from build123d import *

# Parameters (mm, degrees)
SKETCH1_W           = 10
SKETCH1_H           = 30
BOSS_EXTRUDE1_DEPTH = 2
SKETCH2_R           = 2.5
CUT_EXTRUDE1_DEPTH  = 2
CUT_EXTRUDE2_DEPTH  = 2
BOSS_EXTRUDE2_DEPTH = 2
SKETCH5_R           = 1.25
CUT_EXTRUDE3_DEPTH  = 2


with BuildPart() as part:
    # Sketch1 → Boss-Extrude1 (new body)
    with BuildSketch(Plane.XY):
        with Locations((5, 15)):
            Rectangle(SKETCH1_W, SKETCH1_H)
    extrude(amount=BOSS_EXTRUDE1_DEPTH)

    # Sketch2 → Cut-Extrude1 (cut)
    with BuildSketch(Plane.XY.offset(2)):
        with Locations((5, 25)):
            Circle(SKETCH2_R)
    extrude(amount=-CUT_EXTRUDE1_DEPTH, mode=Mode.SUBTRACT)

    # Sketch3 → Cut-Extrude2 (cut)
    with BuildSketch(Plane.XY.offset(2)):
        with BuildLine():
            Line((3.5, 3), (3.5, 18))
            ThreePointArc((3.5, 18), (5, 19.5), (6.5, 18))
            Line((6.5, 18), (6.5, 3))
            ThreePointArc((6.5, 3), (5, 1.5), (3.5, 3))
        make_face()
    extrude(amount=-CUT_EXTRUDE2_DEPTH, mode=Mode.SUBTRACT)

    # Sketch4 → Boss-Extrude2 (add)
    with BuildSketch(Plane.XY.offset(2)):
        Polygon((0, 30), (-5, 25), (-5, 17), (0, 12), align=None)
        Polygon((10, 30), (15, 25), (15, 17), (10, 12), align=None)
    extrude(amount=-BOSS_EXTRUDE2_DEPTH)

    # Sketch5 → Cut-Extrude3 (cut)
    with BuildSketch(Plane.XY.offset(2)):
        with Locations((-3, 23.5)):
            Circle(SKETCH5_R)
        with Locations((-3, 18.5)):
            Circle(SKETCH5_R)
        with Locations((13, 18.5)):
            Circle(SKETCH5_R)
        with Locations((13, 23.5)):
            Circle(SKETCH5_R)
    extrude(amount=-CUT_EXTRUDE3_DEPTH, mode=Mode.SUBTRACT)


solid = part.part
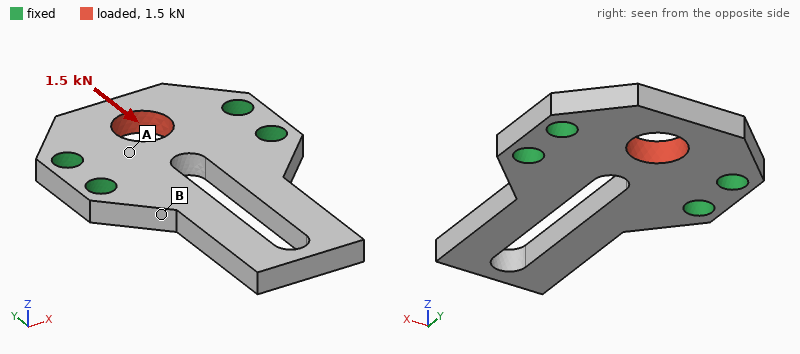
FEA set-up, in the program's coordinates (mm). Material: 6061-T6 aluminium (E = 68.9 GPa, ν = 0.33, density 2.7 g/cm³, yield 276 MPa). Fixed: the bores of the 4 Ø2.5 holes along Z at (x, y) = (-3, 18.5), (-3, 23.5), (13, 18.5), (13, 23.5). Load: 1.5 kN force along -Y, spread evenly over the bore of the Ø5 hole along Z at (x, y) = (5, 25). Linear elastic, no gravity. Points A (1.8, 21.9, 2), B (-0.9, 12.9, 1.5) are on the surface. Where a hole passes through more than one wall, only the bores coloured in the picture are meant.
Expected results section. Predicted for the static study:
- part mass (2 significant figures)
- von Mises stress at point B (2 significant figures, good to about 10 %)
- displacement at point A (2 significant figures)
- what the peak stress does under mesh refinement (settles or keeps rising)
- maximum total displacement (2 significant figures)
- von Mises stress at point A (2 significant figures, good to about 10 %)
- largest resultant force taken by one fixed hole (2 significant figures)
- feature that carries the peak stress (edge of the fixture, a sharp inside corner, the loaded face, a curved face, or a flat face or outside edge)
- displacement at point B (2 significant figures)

1.8 g
18 MPa
5.7 µm
keeps rising
13 µm
55 MPa
450 N
edge of the fixture
5.1 µm
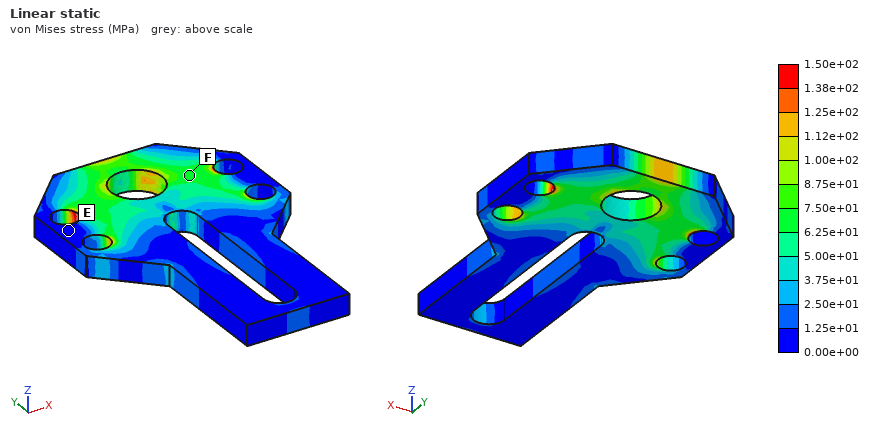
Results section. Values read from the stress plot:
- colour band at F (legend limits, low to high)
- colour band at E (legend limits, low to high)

6.25e+01 to 7.50e+01 MPa
0.00e+00 to 1.25e+01 MPa
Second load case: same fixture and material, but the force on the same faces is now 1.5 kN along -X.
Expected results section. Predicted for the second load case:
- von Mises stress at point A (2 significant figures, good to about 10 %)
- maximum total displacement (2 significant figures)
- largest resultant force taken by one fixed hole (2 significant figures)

39 MPa
9.5 µm
630 N
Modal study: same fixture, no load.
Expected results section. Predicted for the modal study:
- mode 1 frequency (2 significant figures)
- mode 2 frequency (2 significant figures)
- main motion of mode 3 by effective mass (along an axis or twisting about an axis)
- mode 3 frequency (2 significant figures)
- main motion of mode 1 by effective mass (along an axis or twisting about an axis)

5200 Hz
16 kHz
along X
18 kHz
along Z
